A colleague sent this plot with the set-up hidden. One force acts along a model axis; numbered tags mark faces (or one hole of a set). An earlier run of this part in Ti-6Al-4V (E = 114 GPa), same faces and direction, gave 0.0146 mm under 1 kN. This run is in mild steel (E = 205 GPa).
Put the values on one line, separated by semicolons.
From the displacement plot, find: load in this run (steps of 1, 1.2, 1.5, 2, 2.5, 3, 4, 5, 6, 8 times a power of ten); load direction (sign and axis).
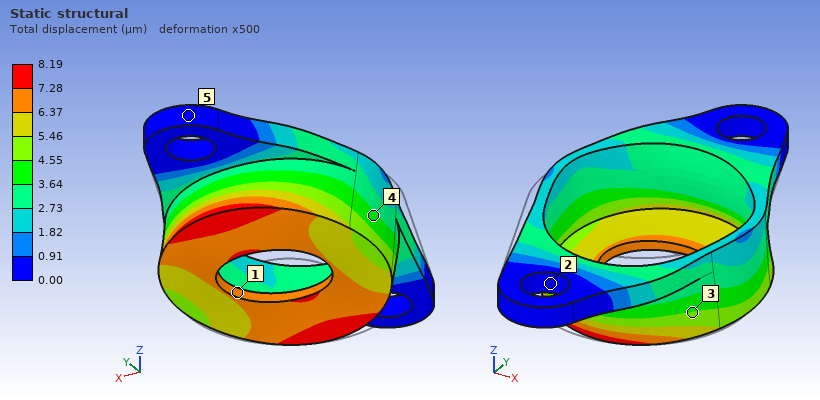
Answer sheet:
1 kN; +Y
